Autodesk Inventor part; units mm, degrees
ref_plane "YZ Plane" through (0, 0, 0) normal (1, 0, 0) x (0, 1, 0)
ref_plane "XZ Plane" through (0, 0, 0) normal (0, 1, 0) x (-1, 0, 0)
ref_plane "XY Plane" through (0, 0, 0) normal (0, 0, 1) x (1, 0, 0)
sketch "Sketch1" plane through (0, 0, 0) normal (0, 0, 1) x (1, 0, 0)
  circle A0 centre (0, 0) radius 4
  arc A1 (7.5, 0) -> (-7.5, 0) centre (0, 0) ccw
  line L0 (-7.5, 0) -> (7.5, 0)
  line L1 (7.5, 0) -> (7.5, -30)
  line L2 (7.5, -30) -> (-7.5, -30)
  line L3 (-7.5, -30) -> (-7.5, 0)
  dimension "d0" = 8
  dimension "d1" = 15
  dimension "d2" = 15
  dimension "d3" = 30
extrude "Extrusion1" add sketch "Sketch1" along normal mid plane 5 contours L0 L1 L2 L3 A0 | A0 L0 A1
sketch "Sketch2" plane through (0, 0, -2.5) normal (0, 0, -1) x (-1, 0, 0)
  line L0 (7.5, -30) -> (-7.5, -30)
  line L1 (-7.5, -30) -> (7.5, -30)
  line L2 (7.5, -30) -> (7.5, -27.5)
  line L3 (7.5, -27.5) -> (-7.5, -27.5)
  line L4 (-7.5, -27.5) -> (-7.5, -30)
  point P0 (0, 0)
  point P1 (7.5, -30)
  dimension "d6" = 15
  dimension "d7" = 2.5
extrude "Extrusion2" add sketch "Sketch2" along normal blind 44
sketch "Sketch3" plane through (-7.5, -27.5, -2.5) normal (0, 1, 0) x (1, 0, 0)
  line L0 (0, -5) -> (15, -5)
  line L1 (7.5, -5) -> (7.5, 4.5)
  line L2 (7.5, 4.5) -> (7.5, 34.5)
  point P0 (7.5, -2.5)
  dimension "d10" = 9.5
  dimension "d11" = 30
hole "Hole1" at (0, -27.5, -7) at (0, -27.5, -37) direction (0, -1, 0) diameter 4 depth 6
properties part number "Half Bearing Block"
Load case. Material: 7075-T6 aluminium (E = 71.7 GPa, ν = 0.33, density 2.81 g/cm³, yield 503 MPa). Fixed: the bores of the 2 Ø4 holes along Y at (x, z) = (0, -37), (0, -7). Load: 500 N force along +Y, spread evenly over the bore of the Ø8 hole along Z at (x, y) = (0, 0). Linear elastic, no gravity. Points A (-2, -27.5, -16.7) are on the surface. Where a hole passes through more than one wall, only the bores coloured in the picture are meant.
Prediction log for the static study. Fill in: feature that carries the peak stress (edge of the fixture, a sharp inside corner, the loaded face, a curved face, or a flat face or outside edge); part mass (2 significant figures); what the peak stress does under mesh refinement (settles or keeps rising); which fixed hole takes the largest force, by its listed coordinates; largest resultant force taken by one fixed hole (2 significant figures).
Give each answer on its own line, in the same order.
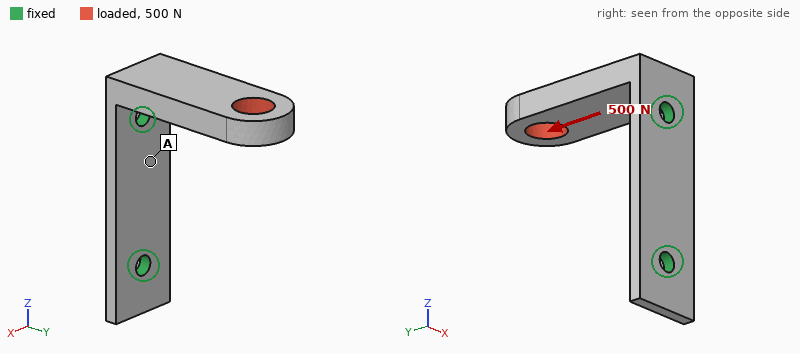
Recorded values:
edge of the fixture
11 g
keeps rising
(0, -7)
510 N
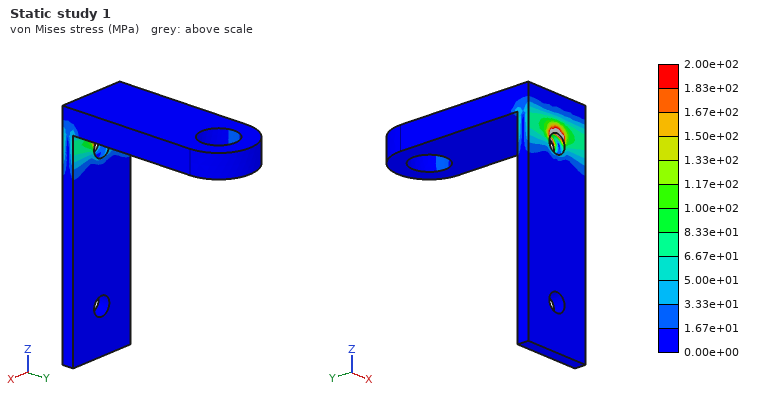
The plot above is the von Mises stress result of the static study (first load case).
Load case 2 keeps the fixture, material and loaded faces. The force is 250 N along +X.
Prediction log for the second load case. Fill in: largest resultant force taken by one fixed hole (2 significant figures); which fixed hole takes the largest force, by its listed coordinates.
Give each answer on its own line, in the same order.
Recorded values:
280 N
(0, -7)
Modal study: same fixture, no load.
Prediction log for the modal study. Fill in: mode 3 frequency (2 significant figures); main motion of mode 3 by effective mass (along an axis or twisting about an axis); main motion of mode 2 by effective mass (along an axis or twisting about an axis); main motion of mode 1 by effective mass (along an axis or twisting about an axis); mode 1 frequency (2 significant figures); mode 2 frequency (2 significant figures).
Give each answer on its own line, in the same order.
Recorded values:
11 kHz
along Y
along X
along Z
1600 Hz
2600 Hz
